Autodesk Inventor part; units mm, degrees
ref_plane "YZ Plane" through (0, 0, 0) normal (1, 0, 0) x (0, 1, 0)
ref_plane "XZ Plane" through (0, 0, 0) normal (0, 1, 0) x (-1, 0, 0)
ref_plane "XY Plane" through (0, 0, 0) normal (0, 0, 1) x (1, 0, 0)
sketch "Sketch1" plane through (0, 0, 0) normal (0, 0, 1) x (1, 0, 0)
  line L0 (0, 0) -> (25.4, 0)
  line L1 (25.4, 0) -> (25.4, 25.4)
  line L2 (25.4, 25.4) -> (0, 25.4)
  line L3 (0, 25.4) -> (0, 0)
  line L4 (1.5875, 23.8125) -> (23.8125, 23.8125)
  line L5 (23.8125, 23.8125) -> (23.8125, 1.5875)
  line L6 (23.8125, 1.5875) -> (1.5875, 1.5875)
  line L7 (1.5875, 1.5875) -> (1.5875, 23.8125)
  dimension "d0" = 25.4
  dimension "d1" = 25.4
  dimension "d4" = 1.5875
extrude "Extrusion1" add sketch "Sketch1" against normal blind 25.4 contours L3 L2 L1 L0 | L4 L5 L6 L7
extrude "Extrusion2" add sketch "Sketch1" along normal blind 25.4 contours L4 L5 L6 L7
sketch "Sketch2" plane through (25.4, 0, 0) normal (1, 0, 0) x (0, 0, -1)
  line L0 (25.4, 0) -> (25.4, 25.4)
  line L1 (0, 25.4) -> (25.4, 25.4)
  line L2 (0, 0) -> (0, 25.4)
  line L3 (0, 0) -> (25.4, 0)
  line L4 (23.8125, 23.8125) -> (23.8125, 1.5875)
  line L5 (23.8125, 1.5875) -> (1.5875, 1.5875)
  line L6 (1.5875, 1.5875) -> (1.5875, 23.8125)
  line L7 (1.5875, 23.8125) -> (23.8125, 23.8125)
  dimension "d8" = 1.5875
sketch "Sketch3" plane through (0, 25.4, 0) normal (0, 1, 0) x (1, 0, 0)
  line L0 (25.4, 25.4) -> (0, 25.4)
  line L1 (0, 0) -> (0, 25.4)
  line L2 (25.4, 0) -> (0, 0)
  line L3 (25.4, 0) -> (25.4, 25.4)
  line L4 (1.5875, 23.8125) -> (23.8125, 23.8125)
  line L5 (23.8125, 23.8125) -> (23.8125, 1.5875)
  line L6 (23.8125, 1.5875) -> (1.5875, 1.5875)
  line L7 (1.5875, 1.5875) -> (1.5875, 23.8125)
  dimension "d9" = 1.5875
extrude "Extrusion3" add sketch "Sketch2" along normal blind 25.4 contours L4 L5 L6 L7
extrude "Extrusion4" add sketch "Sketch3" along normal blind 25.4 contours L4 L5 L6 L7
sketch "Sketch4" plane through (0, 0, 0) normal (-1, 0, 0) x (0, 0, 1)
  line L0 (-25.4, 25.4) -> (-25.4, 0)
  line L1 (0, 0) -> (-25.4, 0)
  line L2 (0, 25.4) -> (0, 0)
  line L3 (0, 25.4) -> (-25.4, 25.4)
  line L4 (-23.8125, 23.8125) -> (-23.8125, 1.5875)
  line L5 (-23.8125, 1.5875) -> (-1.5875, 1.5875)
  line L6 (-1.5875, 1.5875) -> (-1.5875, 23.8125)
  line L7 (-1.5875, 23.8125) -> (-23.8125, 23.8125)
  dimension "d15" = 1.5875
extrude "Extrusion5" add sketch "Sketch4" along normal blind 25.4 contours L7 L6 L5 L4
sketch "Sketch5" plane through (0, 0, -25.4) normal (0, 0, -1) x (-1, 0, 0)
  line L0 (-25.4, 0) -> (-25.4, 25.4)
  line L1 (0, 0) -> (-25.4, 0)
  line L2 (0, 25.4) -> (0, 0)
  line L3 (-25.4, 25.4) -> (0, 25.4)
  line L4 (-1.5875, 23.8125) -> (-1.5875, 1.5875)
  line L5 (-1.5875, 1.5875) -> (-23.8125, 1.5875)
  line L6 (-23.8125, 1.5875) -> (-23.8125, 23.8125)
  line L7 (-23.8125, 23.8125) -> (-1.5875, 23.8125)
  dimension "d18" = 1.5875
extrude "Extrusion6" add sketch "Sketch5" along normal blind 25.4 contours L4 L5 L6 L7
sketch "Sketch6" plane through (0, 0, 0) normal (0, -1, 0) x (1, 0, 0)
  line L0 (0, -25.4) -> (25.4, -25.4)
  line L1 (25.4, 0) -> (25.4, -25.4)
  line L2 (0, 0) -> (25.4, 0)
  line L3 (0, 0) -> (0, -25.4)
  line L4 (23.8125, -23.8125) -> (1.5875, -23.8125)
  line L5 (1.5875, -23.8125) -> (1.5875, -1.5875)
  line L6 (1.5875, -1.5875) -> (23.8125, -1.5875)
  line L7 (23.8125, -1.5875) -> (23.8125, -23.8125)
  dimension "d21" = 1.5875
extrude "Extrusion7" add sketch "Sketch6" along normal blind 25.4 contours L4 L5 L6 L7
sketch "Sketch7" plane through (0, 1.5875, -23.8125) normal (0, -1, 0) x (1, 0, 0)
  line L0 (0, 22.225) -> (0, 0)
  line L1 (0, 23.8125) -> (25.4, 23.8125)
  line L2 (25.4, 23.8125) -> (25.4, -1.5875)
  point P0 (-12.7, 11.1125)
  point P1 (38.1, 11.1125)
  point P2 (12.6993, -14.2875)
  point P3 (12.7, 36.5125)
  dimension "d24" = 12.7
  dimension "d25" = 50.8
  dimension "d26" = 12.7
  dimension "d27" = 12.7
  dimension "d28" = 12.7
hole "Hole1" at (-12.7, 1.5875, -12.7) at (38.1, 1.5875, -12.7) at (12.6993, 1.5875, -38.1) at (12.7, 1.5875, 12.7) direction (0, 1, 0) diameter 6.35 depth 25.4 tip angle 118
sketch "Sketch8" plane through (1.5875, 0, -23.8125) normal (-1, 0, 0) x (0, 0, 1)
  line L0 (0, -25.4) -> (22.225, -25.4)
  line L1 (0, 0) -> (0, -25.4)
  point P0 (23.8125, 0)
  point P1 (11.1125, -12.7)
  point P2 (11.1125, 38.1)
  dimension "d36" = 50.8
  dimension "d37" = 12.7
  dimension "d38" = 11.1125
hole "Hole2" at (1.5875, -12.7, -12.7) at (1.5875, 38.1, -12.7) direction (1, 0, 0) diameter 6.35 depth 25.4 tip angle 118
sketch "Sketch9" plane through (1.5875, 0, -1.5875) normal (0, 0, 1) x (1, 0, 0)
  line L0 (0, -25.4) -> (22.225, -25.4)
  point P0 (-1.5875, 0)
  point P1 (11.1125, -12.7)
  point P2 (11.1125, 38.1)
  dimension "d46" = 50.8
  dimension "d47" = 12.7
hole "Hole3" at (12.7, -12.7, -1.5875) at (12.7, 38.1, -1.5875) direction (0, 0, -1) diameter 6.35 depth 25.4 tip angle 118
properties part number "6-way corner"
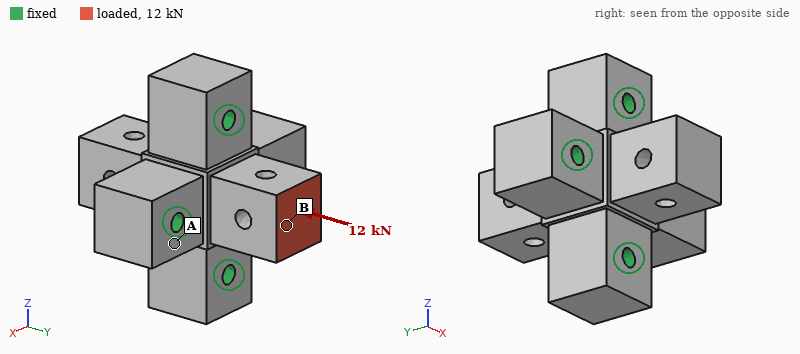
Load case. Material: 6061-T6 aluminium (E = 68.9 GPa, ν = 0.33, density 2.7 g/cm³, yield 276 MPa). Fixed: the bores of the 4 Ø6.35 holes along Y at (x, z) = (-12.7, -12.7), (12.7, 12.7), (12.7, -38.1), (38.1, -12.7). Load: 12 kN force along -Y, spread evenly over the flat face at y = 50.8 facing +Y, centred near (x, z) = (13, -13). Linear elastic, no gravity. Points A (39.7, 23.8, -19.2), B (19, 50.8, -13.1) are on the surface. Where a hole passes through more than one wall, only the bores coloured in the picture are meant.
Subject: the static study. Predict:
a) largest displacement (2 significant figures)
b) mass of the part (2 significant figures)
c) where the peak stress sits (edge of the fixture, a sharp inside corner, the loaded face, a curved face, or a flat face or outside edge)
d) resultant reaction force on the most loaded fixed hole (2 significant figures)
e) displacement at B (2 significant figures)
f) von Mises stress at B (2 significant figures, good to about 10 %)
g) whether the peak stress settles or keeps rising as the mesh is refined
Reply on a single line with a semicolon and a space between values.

20 µm; 230 g; a sharp inside corner; 3.1 kN; 19 µm; 18 MPa; keeps rising
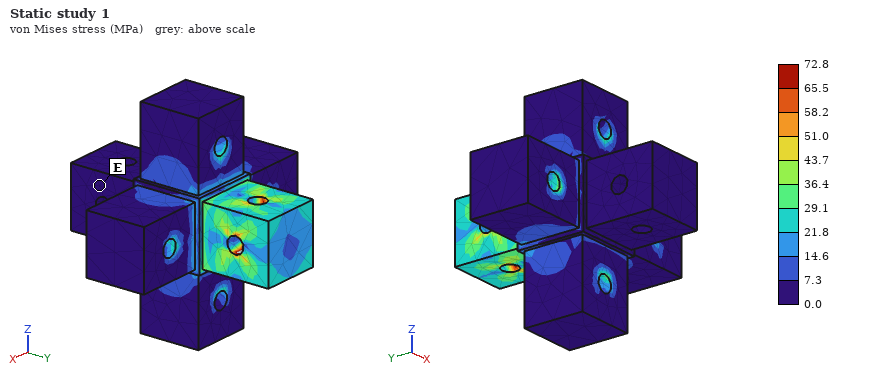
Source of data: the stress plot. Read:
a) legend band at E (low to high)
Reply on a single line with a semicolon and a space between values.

0.0 to 7.3 MPa
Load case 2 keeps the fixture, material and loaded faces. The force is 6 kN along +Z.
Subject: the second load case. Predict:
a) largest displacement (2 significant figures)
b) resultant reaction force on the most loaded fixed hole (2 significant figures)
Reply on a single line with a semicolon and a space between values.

81 µm; 5.2 kN
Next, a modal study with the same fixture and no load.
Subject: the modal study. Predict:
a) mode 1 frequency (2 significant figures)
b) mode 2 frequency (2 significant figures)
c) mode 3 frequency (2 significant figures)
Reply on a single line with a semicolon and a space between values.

13 kHz; 13 kHz; 14 kHz
